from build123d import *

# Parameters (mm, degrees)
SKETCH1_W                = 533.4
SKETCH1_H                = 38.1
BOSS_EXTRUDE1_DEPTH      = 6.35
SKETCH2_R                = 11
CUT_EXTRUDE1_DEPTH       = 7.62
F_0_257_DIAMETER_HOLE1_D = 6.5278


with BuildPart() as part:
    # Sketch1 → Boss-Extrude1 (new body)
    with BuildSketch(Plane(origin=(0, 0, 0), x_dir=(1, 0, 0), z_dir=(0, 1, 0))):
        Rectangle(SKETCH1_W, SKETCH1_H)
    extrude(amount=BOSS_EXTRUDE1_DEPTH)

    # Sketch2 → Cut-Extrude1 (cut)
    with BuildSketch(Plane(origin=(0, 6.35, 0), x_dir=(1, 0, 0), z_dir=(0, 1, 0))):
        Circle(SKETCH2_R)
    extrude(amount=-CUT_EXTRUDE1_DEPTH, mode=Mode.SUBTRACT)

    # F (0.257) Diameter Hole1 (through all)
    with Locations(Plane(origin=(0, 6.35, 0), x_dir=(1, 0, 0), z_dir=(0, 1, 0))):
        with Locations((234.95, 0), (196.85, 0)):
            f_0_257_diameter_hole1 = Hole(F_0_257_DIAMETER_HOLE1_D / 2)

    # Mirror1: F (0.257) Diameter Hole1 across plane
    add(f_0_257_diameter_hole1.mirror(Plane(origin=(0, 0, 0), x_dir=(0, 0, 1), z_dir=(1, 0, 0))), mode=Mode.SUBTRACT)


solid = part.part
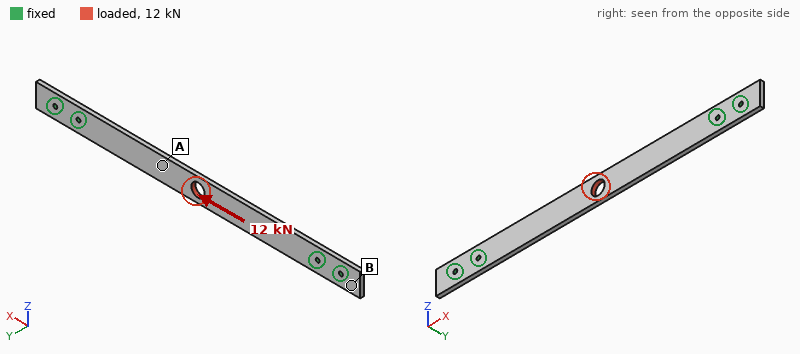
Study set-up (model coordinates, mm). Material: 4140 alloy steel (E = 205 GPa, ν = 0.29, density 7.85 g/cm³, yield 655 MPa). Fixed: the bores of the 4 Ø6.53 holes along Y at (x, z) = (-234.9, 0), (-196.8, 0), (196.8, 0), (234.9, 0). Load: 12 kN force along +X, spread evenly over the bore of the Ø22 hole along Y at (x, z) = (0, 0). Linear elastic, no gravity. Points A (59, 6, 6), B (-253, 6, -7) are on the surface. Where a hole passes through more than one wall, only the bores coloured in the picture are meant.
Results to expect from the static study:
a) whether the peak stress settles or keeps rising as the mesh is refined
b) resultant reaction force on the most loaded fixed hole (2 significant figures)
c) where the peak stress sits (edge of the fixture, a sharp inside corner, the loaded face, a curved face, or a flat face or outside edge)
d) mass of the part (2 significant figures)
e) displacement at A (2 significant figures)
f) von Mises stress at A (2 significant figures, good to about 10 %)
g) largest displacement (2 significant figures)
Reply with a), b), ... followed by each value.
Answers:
a) keeps rising
b) 4.9 kN
c) edge of the fixture
d) 990 g
e) 18 µm
f) 25 MPa
g) 25 µm
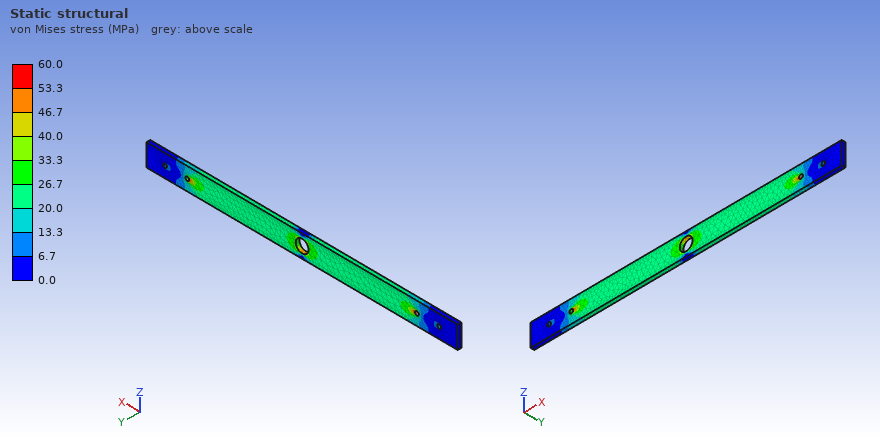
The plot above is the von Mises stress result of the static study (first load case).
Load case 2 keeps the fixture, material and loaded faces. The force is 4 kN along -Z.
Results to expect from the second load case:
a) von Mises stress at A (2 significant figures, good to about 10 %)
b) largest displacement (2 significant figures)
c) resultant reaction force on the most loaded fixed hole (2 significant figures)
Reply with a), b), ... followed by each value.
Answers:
a) 27 MPa
b) 0.30 mm
c) 5.7 kN
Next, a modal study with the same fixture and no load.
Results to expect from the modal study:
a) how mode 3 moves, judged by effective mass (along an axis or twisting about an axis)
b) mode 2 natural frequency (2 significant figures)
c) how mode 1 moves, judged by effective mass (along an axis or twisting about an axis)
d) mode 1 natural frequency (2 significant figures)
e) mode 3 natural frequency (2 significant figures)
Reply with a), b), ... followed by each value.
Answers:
a) along Z
b) 590 Hz
c) along Y
d) 210 Hz
e) 1100 Hz
